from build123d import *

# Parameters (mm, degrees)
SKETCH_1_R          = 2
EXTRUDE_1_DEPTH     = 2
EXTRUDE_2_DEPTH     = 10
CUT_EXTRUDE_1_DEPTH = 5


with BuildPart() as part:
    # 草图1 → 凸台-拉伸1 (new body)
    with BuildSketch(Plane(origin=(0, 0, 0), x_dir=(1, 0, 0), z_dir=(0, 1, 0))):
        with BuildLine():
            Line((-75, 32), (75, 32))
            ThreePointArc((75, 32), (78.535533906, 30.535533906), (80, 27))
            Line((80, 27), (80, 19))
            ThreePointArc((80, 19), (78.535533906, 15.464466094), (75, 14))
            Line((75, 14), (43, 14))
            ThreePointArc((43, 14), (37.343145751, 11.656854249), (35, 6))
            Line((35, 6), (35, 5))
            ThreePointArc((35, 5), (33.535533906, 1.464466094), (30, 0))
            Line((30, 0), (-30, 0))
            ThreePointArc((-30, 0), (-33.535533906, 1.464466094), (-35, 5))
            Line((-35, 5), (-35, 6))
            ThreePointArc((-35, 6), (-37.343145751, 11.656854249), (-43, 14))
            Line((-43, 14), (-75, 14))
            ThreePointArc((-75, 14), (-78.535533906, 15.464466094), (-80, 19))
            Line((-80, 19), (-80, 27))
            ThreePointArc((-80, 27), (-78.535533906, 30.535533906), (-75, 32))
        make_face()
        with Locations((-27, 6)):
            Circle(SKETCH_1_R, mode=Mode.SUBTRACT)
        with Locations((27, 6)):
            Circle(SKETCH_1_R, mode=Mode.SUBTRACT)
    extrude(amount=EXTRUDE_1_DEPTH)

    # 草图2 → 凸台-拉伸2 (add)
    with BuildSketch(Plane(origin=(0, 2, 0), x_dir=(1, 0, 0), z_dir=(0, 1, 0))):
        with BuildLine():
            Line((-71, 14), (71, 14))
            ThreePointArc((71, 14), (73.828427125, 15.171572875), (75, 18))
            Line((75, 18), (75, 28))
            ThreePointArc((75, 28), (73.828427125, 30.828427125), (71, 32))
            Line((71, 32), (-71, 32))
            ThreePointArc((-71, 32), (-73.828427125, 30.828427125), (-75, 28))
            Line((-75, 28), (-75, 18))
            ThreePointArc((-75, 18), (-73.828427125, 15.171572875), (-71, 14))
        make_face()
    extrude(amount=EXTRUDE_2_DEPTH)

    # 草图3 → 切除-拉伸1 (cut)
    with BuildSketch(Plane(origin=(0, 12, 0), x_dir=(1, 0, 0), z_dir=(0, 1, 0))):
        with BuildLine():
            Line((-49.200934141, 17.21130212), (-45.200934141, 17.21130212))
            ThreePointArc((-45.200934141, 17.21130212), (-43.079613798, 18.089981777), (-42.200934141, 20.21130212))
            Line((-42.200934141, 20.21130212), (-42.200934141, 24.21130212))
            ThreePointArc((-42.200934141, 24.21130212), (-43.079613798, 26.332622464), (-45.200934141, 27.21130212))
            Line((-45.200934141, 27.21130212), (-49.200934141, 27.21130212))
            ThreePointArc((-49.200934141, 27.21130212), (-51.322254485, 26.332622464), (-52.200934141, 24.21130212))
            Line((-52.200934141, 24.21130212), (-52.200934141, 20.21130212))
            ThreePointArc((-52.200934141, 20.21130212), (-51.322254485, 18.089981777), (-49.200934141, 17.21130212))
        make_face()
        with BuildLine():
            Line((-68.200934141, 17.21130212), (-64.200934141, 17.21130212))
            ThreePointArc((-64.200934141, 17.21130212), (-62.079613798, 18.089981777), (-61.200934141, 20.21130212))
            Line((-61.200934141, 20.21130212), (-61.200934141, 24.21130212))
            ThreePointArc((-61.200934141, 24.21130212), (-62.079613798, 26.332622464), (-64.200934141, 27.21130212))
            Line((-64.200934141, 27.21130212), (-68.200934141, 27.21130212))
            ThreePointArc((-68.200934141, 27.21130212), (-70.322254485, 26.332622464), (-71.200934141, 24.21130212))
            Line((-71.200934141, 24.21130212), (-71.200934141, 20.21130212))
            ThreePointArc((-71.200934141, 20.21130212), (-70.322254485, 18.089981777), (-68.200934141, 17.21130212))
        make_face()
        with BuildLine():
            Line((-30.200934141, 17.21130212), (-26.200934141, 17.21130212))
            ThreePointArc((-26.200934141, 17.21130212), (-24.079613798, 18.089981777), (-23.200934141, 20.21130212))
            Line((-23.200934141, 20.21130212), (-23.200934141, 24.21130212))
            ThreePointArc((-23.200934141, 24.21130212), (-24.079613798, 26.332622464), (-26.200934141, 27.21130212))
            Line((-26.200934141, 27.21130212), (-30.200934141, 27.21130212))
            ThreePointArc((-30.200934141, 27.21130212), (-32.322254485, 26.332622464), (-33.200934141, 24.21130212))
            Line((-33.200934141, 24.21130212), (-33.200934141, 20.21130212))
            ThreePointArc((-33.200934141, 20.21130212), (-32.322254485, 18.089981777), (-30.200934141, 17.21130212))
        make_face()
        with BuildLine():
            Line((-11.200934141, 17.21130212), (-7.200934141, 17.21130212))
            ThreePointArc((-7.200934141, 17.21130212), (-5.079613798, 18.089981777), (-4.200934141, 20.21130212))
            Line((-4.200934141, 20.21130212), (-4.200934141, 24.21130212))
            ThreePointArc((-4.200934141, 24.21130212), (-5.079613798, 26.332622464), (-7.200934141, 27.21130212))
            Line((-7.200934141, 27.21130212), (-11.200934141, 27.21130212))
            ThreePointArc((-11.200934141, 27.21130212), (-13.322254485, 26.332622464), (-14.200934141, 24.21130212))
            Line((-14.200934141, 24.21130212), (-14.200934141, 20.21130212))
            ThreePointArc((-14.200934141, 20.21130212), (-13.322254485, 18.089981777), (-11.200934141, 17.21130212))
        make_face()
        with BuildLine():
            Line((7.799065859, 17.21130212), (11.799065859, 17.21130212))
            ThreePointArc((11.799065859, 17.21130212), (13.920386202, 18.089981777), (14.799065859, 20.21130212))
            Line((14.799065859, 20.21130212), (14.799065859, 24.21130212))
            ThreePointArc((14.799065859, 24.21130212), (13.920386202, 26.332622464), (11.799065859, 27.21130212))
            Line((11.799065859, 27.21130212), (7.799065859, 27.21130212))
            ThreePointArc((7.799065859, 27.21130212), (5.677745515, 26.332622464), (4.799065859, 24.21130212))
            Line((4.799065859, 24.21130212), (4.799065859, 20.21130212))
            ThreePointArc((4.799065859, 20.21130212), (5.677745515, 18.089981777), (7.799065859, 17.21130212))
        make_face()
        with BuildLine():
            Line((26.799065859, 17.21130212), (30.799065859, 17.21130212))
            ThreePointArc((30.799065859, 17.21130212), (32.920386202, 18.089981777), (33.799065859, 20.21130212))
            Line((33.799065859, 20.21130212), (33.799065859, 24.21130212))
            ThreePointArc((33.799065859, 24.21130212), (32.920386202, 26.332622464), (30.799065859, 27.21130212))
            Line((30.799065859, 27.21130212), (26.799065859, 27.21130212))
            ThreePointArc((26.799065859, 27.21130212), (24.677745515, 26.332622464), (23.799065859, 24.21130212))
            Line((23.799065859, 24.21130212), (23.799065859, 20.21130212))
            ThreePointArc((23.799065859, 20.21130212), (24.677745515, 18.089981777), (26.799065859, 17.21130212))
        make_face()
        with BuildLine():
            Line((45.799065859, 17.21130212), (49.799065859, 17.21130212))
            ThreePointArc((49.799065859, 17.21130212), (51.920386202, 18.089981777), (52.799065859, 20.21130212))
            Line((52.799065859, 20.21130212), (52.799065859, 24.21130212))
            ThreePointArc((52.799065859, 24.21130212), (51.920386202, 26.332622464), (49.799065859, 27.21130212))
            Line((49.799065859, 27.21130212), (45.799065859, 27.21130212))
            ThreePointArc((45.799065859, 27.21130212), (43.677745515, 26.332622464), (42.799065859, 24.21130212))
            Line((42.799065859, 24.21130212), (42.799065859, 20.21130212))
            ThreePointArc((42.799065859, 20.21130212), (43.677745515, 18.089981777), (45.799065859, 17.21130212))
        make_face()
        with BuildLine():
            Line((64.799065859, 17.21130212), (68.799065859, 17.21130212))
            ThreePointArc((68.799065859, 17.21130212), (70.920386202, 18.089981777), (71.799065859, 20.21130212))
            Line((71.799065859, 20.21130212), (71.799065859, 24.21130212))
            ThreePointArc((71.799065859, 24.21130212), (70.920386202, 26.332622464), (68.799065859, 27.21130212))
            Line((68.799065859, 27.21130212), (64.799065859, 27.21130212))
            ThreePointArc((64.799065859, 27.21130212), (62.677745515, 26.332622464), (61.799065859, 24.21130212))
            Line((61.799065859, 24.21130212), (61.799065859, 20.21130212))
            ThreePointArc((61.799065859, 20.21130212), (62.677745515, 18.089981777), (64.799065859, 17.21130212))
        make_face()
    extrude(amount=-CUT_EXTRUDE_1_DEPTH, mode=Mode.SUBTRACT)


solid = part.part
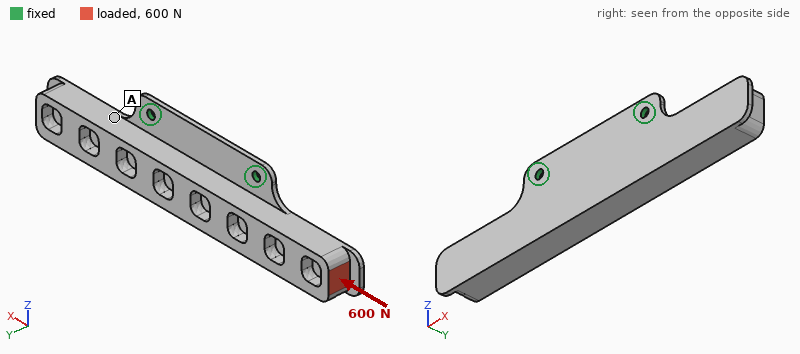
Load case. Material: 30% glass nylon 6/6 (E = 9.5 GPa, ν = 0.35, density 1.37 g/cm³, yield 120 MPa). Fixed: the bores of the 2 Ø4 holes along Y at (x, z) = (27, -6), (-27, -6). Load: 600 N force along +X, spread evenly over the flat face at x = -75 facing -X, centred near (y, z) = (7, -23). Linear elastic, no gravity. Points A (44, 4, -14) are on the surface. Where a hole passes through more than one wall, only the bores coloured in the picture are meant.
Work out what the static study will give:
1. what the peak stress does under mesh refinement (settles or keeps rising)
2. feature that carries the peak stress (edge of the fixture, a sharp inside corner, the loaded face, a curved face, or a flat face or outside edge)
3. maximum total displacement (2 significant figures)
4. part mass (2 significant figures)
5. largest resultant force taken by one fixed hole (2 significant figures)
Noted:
keeps rising
edge of the fixture
0.29 mm
42 g
360 N
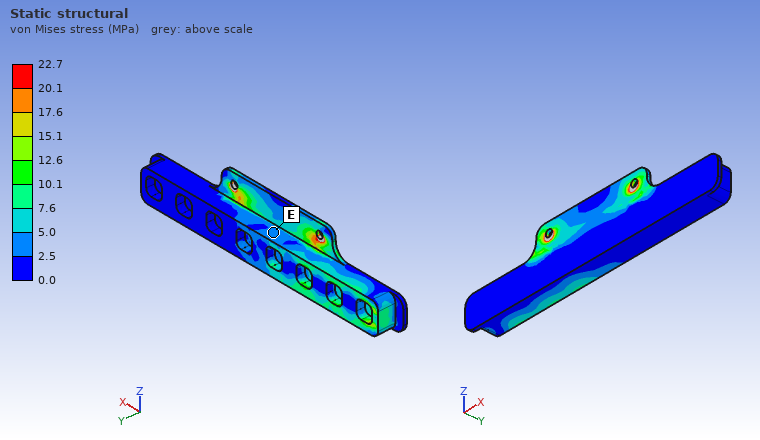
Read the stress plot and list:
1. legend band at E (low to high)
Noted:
2.5 to 5.0 MPa
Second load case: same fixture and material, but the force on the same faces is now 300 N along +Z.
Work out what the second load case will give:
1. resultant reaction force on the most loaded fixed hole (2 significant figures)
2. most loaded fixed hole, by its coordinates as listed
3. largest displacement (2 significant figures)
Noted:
600 N
(-27, -6)
1.6 mm
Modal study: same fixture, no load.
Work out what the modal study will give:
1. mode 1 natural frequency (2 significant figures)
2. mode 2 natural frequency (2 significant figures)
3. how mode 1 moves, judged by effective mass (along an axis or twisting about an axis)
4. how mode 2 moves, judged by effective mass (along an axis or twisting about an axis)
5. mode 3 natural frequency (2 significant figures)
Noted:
330 Hz
700 Hz
along Y
twisting about Z
1300 Hz
